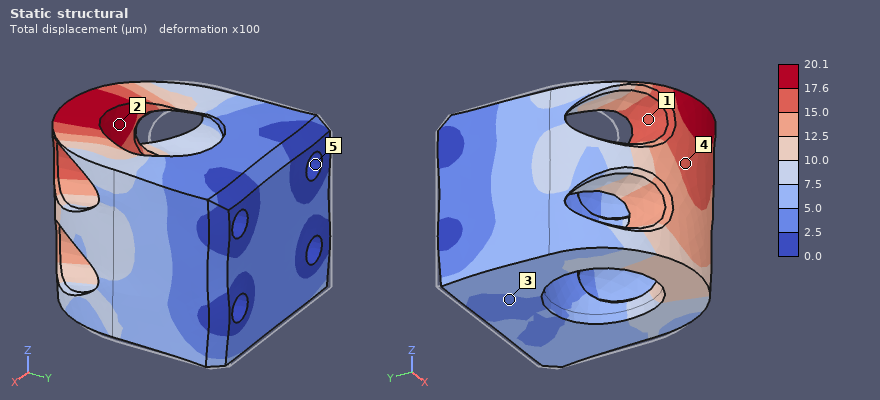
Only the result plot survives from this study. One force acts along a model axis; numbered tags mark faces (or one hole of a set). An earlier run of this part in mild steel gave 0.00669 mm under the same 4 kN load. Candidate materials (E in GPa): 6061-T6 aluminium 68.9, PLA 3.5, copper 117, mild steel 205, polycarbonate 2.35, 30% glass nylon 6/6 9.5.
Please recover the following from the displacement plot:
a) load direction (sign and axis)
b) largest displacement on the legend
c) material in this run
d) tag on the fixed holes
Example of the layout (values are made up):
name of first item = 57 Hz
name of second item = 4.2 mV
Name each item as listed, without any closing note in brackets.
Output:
load direction = -Y
largest displacement on the legend = 20.1 µm
material in this run = 6061-T6 aluminium
tag on the fixed holes = 5
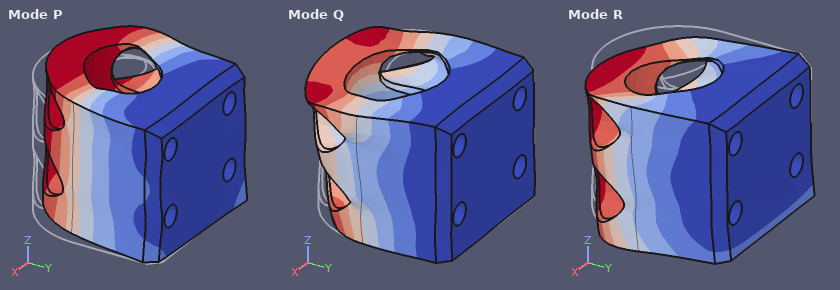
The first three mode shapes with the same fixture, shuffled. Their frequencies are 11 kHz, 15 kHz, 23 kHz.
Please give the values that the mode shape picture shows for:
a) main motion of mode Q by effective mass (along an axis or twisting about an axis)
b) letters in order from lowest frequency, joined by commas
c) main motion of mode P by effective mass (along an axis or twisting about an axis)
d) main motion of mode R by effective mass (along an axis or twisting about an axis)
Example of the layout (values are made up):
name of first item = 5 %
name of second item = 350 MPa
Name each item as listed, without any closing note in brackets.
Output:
main motion of mode Q by effective mass = twisting about Y
letters in order from lowest frequency, joined by commas = R, P, Q
main motion of mode P by effective mass = along X
main motion of mode R by effective mass = along Z
